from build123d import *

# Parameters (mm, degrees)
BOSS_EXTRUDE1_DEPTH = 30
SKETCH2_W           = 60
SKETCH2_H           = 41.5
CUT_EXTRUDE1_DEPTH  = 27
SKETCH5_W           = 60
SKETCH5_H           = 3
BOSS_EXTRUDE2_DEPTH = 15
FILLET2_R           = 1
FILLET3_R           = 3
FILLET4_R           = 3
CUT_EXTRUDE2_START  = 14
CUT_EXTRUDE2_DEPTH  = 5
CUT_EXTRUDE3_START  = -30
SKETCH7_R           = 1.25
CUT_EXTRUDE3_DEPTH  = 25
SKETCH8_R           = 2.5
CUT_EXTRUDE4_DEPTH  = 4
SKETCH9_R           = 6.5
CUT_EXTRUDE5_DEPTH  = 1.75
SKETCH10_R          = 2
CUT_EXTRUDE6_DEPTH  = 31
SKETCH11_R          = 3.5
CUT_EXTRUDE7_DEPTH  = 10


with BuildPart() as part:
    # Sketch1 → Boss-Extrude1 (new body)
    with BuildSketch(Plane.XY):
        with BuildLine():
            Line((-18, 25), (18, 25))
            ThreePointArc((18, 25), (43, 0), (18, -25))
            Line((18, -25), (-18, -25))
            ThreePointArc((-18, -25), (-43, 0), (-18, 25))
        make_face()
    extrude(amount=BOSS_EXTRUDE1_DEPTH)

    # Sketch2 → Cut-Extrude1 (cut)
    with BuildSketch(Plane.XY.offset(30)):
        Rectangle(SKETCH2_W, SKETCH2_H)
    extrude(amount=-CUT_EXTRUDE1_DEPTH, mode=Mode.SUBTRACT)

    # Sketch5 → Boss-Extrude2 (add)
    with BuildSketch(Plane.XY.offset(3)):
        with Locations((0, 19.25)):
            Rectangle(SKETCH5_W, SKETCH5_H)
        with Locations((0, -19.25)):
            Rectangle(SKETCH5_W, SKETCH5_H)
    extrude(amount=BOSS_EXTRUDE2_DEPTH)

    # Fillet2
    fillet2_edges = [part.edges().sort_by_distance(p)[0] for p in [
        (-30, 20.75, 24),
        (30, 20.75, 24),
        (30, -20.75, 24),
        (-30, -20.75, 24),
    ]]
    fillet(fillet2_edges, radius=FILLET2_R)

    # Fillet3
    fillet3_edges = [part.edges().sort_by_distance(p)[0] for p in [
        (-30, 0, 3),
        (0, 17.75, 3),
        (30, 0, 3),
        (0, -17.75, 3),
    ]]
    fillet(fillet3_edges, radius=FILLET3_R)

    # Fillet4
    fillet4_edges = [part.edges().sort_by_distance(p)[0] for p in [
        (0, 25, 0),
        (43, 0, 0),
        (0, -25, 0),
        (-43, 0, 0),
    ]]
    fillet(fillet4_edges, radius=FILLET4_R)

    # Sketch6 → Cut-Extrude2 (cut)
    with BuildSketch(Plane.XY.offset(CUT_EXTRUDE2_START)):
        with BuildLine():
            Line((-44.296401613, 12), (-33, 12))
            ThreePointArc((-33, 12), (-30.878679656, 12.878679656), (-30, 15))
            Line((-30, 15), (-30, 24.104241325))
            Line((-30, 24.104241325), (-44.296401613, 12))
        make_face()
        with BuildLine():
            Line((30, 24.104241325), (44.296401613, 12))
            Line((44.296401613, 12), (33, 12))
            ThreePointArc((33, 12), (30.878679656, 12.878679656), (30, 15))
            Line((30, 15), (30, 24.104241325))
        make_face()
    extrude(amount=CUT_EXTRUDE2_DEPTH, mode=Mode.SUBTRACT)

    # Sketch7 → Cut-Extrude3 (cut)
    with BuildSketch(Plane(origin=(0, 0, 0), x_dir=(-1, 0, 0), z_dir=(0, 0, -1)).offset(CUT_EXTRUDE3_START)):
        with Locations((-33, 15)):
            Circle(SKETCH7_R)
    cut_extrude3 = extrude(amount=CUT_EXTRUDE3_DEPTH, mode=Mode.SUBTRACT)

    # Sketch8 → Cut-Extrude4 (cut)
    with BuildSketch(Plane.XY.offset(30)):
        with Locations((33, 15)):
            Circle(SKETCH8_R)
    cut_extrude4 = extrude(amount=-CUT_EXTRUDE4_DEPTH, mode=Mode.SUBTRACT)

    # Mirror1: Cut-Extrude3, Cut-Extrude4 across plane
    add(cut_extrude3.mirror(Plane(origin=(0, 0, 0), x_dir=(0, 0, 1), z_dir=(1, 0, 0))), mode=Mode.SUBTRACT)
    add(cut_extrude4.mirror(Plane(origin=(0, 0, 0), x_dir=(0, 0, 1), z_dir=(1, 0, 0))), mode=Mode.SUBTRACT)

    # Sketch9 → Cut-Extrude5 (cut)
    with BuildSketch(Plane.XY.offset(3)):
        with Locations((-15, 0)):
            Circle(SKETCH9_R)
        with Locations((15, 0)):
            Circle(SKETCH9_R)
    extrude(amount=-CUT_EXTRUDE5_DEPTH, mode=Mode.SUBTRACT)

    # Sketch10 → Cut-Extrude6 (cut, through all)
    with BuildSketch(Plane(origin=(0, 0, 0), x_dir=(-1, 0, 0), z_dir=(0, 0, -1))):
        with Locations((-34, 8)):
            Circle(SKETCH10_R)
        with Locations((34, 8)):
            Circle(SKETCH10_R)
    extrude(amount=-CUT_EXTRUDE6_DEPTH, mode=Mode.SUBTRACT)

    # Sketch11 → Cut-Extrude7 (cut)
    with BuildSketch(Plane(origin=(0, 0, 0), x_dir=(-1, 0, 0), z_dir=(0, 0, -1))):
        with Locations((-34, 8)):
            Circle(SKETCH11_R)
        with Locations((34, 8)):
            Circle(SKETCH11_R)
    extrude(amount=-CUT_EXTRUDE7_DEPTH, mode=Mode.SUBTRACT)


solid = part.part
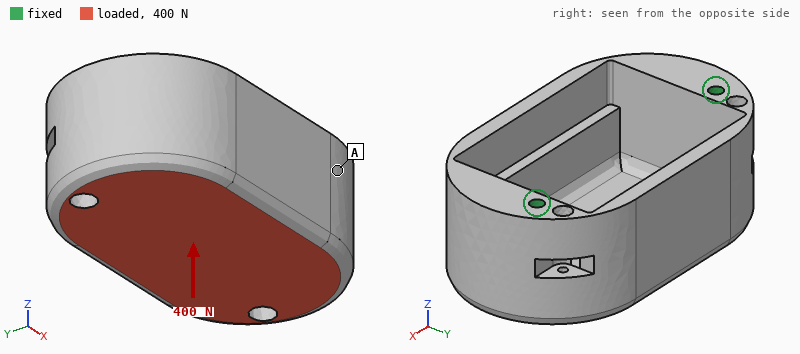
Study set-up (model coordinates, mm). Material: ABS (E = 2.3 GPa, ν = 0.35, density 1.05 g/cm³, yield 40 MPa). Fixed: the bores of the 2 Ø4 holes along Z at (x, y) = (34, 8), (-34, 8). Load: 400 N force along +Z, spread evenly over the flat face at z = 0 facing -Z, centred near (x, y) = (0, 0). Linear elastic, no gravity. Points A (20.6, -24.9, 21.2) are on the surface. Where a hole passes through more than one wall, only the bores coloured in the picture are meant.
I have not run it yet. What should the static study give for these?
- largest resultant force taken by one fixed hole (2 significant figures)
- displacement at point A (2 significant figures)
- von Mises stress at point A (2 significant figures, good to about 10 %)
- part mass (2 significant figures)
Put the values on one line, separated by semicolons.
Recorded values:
200 N; 0.053 mm; 0.64 MPa; 51 g
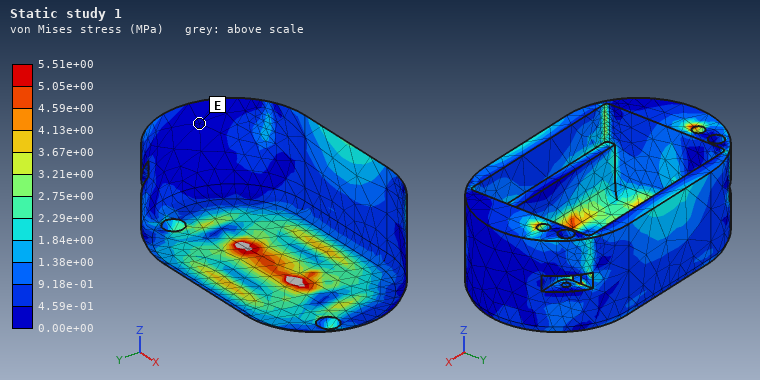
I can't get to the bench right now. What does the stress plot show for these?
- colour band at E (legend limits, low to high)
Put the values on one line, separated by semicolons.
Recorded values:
0.00e+00 to 4.59e-01 MPa
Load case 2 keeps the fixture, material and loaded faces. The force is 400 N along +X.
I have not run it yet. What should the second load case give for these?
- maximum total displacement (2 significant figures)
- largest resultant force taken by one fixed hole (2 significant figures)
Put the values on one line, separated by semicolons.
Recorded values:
54 µm; 210 N
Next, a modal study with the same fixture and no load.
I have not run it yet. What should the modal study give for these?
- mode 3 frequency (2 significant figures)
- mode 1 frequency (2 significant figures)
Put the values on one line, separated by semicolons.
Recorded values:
2000 Hz; 1800 Hz
